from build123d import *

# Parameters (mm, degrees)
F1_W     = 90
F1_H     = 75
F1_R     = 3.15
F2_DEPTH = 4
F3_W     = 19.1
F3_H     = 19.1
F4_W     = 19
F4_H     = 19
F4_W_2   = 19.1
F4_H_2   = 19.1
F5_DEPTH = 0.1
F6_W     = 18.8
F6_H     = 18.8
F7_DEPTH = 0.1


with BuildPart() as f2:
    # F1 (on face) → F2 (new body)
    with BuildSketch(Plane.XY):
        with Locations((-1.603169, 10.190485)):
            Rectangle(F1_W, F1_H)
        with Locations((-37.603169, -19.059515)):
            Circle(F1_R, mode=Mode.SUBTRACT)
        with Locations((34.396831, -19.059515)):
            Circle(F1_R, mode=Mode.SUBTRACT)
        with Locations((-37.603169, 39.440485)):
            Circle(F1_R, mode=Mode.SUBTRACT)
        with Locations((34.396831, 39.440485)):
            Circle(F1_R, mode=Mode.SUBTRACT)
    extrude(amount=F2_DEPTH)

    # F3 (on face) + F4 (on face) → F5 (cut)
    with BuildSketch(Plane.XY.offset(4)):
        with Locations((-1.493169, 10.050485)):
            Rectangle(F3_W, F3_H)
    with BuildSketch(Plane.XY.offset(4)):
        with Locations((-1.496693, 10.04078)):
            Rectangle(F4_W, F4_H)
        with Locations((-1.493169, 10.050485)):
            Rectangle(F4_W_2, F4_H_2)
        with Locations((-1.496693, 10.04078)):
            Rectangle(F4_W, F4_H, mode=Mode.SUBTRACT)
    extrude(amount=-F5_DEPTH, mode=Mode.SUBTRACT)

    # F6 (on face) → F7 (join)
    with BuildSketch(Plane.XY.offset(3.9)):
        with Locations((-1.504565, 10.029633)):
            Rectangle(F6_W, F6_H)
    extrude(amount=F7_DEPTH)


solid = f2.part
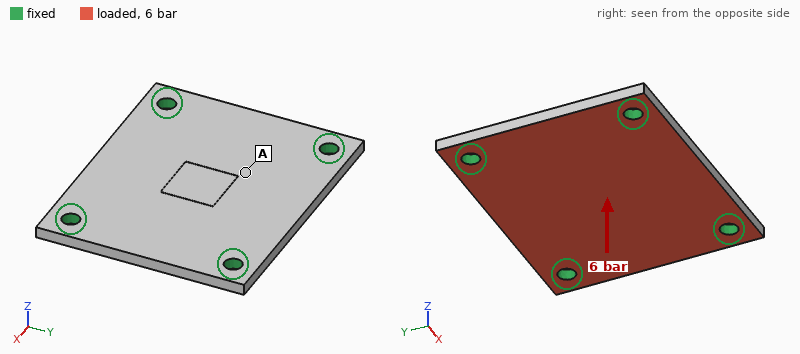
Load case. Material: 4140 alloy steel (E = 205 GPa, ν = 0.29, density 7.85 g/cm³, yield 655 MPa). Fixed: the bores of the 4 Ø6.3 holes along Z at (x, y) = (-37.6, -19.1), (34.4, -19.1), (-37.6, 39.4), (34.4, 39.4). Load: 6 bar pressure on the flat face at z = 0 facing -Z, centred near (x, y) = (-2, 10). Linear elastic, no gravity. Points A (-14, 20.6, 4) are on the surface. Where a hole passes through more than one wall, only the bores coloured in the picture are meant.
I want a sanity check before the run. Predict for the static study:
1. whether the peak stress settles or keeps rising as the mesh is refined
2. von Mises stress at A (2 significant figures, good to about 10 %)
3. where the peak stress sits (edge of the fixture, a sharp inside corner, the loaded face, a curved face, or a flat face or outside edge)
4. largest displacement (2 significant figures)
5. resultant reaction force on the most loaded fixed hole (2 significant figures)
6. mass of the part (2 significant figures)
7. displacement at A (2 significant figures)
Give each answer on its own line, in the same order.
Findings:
keeps rising
36 MPa
edge of the fixture
61 µm
990 N
210 g
50 µm
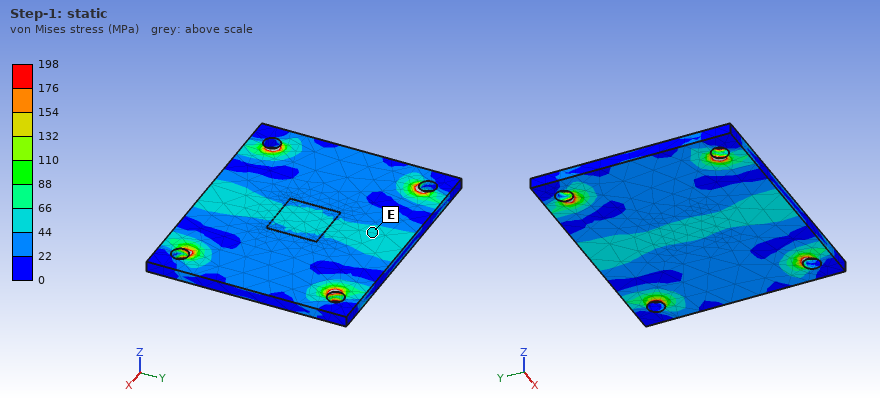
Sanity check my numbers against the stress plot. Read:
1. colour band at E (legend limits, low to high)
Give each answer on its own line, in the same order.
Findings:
44 to 66 MPa
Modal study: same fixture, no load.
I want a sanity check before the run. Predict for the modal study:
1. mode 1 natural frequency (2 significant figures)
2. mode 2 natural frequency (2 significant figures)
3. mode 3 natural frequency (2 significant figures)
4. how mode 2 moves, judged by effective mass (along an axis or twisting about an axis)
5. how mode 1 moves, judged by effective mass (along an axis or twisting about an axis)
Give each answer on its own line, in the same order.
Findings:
3400 Hz
5000 Hz
6300 Hz
twisting about X
along Z
